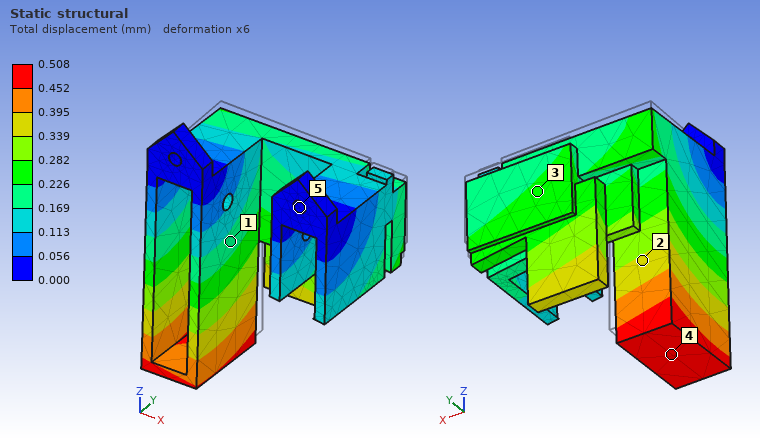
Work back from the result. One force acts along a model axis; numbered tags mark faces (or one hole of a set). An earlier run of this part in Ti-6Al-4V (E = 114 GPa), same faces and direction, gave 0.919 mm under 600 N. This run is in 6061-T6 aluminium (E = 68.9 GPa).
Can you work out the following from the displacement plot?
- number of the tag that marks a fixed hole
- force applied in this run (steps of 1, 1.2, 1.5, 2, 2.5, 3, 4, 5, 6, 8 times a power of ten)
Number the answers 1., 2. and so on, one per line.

1. 5
2. 200 N
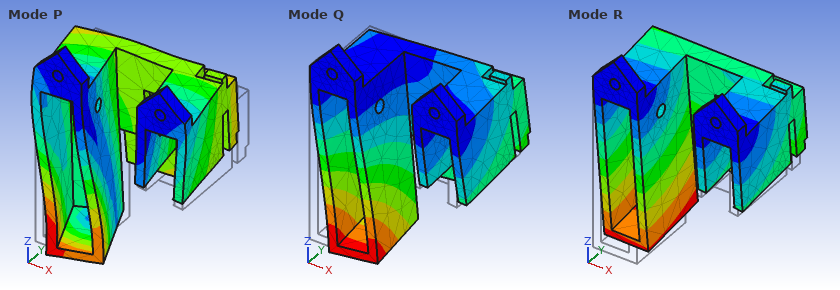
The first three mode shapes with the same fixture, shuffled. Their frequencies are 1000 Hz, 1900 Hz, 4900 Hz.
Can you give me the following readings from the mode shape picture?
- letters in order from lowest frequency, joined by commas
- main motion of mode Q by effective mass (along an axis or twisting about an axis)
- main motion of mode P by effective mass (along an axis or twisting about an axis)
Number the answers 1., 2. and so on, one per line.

1. R, Q, P
2. along X
3. along X
